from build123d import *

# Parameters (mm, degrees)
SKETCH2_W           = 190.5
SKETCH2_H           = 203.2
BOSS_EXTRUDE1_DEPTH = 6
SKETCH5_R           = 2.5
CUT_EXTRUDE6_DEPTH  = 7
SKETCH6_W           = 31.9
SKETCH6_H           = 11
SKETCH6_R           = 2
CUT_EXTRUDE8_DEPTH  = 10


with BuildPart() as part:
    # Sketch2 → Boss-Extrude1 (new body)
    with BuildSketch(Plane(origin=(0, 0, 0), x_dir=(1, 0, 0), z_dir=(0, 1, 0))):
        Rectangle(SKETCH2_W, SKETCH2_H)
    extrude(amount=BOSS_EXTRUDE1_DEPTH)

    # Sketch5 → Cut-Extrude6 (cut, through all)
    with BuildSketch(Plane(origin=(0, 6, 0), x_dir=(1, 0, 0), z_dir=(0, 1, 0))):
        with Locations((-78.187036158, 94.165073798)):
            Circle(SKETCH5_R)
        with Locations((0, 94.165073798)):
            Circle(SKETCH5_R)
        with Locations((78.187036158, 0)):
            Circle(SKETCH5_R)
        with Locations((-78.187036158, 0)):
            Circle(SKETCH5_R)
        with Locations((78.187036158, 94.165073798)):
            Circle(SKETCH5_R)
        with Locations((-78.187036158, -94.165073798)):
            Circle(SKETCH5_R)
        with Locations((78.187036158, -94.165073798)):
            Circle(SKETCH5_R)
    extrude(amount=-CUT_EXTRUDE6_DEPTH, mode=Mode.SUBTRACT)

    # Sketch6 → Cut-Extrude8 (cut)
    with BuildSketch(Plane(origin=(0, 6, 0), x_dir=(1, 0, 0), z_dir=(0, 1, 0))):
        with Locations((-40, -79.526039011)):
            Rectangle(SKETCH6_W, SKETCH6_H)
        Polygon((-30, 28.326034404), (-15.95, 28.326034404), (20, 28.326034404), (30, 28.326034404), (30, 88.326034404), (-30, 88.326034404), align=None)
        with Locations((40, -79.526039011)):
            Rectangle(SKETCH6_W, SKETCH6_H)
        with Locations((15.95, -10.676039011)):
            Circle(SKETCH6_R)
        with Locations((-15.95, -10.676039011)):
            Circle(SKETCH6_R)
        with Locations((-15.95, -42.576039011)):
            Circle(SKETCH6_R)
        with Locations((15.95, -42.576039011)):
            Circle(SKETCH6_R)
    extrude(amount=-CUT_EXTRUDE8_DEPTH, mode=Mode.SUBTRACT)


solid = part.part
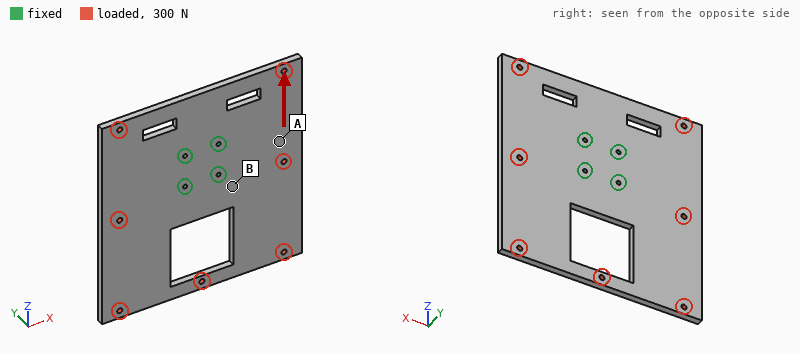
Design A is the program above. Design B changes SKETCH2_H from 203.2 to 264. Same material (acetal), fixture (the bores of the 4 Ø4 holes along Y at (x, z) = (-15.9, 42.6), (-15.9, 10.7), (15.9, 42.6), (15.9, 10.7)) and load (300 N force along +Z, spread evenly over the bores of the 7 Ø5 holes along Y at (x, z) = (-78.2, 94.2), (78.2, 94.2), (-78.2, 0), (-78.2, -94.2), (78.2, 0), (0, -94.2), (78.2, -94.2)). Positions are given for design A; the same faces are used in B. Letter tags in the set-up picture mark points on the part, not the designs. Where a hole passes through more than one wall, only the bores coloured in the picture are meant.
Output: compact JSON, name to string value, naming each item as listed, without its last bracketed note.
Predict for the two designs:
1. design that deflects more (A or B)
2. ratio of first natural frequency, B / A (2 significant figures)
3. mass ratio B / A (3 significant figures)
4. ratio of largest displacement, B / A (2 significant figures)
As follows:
{"design that deflects more": "A", "ratio of first natural frequency, B / A": "0.61", "mass ratio B / A": "1.34", "ratio of largest displacement, B / A": "0.44"}
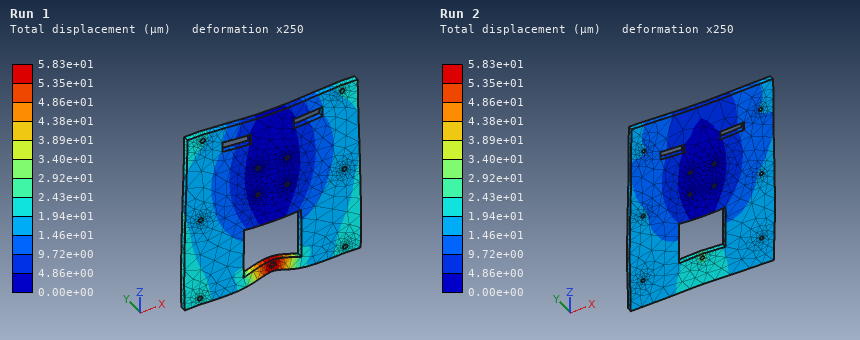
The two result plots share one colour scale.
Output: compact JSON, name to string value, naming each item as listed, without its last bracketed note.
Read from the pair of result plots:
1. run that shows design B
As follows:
{"run that shows design B": "Run 2"}
